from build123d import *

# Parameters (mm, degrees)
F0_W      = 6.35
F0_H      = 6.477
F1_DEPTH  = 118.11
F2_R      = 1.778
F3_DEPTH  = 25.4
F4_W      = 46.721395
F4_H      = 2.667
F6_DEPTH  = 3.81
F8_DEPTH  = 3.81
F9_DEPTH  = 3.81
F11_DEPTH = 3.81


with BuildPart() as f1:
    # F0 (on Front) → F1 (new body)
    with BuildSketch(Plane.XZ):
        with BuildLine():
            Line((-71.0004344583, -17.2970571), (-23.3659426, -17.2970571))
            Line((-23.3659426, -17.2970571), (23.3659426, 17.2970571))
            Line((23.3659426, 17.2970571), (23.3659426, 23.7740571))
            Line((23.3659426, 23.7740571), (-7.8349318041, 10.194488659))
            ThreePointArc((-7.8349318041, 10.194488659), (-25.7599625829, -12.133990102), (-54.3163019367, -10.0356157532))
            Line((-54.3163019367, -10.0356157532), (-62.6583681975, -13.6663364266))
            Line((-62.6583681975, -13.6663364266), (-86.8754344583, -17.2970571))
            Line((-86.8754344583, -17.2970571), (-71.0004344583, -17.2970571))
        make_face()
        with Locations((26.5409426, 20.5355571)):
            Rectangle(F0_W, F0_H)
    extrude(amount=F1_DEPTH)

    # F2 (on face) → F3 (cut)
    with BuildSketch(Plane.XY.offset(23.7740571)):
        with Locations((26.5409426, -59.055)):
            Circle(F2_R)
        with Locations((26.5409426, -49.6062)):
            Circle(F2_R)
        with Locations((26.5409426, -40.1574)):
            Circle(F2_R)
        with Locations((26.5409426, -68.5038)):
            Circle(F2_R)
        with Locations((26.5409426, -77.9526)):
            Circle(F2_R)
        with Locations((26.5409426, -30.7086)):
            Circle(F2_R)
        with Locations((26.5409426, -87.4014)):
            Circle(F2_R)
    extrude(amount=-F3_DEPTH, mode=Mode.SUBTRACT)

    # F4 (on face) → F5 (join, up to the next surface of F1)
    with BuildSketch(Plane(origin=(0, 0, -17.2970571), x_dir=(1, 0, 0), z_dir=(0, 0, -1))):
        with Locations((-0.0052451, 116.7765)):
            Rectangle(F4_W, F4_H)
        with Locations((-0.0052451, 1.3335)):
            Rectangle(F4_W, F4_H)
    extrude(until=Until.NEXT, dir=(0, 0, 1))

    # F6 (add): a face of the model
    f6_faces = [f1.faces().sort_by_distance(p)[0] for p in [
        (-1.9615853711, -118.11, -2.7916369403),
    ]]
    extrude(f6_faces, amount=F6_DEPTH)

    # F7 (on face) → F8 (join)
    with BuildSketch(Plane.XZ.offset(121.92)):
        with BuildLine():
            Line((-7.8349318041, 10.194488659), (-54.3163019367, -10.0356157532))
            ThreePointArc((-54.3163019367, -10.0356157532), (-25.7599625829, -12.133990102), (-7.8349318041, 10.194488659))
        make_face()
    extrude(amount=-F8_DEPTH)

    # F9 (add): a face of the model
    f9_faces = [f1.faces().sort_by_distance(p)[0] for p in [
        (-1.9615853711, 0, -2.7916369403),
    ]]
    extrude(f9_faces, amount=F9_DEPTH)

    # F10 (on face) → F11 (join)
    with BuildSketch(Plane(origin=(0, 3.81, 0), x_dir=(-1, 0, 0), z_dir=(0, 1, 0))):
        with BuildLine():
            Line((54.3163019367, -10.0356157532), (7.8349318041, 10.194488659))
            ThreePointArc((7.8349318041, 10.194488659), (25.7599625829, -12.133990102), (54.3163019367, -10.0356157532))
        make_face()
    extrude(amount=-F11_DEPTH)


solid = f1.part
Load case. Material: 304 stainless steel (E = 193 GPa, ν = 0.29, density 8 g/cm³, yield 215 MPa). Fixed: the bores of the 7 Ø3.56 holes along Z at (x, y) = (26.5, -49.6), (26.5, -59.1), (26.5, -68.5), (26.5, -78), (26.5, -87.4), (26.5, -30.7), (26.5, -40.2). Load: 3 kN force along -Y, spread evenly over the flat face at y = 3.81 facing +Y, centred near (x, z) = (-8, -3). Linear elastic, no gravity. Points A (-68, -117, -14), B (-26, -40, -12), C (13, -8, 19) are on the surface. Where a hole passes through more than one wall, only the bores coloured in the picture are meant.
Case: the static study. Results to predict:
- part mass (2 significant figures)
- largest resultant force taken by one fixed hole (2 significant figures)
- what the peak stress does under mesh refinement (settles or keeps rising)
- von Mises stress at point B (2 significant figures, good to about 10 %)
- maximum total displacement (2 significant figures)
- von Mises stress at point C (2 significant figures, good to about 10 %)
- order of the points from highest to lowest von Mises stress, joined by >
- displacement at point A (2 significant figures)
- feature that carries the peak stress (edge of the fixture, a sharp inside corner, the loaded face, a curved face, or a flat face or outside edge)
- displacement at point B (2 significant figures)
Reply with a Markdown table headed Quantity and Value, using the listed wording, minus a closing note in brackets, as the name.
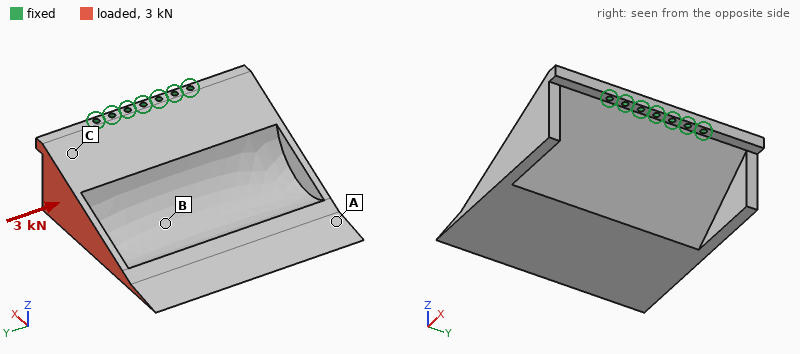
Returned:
| Quantity | Value |
|---|---|
| part mass | 840 g |
| largest resultant force taken by one fixed hole | 1.7 kN |
| what the peak stress does under mesh refinement | keeps rising |
| von Mises stress at point B | 6.9 MPa |
| maximum total displacement | 44 µm |
| von Mises stress at point C | 14 MPa |
| order of the points from highest to lowest von Mises stress, joined by > | C > B > A |
| displacement at point A | 12 µm |
| feature that carries the peak stress | edge of the fixture |
| displacement at point B | 9.0 µm |
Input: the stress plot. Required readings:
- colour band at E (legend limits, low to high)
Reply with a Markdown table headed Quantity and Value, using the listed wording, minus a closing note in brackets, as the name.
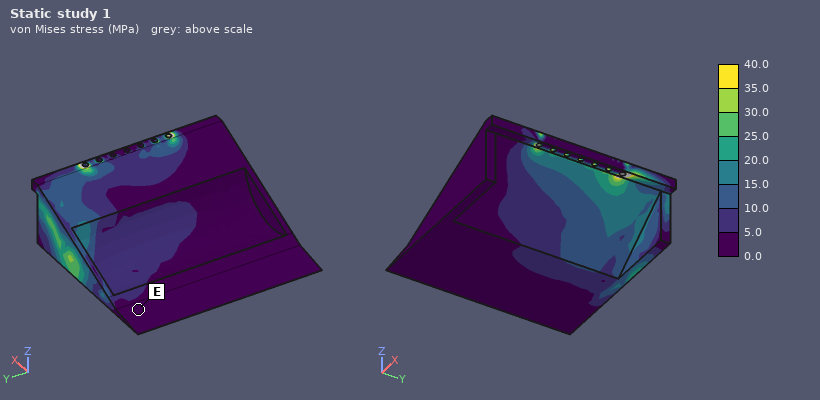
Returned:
| Quantity | Value |
|---|---|
| colour band at E | 0.0 to 5.0 MPa |
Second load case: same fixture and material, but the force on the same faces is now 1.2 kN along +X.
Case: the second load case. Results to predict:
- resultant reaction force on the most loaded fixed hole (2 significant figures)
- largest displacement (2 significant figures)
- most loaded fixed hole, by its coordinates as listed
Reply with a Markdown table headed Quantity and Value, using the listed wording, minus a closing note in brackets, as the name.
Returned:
| Quantity | Value |
|---|---|
| resultant reaction force on the most loaded fixed hole | 1.7 kN |
| largest displacement | 0.21 mm |
| most loaded fixed hole, by its coordinates as listed | (26.5, -30.7) |
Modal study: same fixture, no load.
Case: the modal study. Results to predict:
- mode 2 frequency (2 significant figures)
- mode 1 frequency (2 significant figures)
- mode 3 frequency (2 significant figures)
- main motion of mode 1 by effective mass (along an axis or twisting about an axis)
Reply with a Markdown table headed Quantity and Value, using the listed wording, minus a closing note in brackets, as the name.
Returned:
| Quantity | Value |
|---|---|
| mode 2 frequency | 930 Hz |
| mode 1 frequency | 540 Hz |
| mode 3 frequency | 1800 Hz |
| main motion of mode 1 by effective mass | along Z |
